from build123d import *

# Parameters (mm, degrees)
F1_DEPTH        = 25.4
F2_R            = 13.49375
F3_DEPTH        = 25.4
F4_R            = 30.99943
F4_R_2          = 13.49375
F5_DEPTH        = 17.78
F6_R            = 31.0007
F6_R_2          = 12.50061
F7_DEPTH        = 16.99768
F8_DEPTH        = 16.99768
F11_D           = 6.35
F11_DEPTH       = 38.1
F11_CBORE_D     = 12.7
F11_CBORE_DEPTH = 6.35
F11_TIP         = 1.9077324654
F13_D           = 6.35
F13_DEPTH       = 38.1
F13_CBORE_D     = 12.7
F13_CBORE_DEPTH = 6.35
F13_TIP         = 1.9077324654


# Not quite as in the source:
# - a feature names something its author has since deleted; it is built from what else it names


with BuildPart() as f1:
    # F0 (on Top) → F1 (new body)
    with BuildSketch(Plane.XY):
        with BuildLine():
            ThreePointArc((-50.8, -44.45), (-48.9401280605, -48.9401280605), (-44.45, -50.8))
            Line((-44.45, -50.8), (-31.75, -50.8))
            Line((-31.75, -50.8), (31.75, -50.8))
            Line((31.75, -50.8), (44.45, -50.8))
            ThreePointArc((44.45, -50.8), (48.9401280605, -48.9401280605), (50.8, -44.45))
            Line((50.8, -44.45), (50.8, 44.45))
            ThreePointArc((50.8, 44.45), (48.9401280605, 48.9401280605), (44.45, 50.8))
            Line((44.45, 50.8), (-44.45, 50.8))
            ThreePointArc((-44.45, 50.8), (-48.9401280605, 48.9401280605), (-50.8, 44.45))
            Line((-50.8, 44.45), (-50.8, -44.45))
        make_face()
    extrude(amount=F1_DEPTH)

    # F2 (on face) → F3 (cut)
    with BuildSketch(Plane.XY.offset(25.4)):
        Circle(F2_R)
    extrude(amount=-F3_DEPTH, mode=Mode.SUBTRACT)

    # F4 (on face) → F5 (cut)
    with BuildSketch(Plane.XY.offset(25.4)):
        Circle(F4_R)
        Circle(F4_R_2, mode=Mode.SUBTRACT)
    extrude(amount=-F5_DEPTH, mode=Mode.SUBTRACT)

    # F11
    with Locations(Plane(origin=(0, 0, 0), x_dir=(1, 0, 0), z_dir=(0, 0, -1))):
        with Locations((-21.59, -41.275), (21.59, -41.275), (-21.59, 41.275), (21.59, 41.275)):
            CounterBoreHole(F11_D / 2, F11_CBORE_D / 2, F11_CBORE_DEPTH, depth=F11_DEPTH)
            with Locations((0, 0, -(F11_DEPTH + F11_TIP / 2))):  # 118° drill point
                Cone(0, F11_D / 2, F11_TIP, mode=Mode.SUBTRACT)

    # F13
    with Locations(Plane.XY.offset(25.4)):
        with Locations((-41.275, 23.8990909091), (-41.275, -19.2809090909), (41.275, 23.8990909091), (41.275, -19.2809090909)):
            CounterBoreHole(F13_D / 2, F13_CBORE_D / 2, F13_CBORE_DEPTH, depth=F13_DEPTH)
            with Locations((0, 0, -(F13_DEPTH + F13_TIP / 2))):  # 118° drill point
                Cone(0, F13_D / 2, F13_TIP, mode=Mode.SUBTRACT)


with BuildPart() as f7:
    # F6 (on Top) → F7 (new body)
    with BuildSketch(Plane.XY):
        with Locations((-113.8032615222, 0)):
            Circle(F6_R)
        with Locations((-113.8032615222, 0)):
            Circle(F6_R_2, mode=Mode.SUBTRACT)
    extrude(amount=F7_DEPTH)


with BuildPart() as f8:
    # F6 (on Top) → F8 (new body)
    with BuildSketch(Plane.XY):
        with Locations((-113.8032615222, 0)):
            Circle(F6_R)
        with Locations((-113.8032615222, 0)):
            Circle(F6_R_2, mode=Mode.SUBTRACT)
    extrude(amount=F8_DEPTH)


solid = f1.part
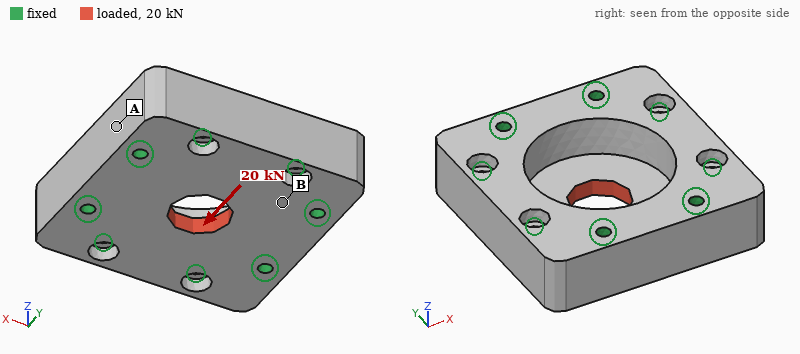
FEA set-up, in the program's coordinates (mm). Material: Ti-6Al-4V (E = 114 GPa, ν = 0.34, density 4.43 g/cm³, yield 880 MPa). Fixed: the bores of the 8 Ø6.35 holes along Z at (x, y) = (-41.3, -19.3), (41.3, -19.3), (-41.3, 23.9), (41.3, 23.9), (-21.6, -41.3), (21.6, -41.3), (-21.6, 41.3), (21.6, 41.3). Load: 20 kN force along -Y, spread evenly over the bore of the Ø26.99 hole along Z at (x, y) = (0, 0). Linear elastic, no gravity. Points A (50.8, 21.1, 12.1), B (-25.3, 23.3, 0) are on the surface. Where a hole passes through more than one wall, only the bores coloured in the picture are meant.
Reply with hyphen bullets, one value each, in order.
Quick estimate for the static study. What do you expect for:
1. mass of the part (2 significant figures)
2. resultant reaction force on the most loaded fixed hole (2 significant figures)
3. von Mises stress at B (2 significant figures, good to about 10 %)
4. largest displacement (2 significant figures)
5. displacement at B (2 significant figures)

- 850 g
- 3.5 kN
- 16 MPa
- 9.8 µm
- 2.7 µm
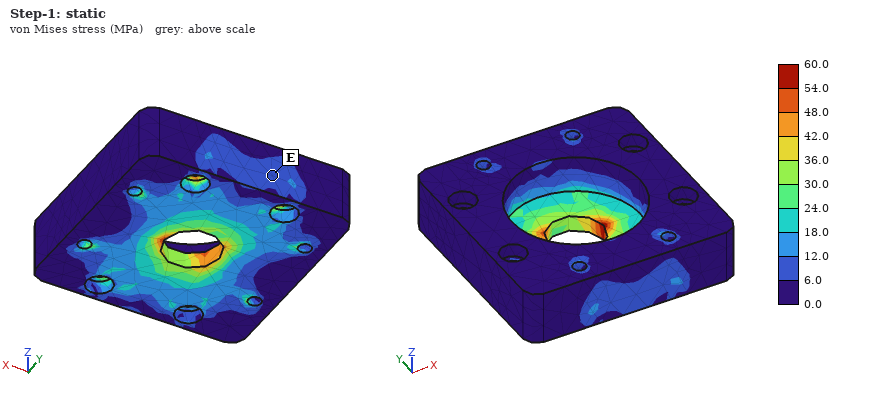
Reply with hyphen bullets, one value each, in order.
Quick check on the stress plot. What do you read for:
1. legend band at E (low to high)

- 6.0 to 12.0 MPa
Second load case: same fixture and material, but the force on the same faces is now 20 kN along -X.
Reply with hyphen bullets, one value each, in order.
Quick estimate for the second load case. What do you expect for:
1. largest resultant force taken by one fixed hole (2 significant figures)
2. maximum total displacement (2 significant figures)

- 4.3 kN
- 8.3 µm
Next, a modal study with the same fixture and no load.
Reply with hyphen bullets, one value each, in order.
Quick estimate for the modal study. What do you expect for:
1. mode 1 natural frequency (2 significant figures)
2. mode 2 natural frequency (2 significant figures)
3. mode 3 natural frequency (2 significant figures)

- 16 kHz
- 19 kHz
- 20 kHz
